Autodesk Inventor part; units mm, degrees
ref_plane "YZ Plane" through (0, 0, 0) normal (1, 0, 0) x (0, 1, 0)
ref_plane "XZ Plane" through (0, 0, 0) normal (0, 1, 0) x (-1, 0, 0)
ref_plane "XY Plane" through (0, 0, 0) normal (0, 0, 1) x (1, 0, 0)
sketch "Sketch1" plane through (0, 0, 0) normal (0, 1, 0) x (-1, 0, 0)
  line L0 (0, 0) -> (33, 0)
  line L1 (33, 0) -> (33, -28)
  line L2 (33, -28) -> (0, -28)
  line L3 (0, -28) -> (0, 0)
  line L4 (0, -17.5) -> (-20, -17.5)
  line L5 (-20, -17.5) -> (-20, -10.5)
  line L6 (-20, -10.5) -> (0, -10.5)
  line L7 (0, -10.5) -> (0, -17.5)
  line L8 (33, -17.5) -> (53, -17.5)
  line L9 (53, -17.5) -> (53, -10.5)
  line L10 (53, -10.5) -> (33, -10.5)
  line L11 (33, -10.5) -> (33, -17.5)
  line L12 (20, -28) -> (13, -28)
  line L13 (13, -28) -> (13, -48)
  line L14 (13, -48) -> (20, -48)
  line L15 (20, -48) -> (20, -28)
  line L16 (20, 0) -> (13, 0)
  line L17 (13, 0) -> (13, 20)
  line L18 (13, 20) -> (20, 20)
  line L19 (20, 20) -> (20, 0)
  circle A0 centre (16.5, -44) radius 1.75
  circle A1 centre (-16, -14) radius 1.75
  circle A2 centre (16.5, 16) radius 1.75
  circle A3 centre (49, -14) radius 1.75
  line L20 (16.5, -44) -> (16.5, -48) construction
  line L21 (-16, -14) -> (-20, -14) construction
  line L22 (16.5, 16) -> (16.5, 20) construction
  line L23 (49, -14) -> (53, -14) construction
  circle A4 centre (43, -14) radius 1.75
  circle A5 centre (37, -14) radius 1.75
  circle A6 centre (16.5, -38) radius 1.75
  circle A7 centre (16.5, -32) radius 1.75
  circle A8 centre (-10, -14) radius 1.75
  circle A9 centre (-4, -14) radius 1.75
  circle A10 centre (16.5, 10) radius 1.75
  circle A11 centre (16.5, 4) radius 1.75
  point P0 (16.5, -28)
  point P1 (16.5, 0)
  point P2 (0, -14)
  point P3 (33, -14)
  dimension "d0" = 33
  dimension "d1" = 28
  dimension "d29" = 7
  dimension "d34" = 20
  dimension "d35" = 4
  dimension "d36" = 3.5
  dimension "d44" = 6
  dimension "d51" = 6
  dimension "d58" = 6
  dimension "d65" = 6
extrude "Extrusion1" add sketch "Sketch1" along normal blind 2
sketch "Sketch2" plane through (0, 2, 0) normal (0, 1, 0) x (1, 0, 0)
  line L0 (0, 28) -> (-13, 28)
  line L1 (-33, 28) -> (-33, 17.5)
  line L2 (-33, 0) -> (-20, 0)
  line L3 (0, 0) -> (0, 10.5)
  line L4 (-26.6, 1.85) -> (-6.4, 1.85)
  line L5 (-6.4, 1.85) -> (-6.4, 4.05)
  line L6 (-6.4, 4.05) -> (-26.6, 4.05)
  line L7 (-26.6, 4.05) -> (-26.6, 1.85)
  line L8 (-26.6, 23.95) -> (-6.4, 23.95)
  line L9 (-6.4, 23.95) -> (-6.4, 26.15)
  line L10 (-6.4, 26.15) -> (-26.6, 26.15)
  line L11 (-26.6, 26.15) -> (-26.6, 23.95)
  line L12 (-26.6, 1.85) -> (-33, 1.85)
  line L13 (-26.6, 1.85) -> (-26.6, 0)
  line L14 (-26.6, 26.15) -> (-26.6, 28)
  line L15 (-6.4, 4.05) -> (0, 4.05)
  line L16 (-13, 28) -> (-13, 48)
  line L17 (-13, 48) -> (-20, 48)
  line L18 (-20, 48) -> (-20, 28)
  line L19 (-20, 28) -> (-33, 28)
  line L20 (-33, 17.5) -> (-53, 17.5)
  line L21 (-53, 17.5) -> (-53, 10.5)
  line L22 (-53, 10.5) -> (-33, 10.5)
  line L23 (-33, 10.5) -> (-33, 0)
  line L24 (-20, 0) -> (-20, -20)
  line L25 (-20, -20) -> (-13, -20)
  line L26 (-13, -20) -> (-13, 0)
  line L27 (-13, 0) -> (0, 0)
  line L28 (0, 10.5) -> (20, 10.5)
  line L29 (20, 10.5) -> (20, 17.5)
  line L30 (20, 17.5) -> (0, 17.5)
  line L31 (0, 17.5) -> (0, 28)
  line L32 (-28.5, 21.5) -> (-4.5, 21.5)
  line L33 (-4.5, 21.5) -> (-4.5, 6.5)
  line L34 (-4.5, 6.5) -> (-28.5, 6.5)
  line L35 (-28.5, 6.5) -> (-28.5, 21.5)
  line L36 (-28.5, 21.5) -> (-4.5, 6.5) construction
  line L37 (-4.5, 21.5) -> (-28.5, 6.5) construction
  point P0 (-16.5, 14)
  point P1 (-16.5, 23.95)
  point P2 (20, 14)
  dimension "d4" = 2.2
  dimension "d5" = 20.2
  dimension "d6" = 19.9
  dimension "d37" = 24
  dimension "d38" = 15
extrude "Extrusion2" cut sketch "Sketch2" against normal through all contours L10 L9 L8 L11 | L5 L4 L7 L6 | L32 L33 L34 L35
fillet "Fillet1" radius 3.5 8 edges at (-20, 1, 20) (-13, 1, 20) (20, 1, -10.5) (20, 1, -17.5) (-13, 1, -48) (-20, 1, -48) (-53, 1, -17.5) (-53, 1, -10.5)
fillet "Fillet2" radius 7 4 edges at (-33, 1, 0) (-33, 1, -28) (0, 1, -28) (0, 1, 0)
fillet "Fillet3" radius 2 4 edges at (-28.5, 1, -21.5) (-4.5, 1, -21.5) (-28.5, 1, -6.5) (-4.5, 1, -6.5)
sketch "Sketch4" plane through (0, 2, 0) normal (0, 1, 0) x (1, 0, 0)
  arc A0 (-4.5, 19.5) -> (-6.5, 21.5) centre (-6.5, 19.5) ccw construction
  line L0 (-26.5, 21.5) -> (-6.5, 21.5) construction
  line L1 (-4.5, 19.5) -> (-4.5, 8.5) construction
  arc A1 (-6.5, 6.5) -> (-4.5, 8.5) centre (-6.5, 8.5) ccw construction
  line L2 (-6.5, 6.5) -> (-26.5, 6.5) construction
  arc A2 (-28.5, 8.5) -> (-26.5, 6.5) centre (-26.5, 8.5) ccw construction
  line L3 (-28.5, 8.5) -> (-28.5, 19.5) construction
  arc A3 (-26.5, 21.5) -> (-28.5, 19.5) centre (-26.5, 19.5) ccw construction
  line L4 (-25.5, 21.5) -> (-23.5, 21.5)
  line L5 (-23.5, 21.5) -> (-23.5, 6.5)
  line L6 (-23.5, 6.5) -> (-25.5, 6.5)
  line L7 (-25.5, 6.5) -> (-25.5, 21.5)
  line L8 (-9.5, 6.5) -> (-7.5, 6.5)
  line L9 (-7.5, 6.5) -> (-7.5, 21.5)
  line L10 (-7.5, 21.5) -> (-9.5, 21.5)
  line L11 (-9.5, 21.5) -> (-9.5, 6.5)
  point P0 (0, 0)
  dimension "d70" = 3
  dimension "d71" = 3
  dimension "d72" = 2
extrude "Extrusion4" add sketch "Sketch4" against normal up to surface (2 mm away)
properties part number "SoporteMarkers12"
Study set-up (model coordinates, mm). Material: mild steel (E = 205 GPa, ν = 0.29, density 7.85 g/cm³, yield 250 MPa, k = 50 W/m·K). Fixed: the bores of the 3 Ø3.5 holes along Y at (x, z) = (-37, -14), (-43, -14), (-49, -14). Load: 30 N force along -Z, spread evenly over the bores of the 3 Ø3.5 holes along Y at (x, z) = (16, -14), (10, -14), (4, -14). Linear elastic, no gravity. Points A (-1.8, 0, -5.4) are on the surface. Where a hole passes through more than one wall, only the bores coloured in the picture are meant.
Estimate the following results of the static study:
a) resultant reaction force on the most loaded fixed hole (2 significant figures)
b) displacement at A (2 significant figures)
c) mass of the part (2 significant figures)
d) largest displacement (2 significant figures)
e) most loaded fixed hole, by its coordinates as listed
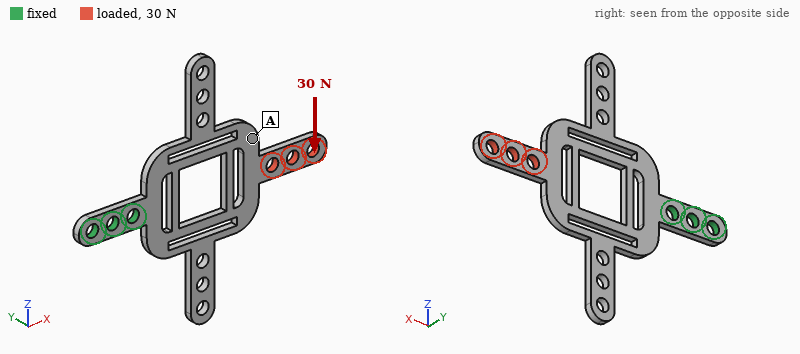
72 N
57 µm
14 g
87 µm
(-37, -14)
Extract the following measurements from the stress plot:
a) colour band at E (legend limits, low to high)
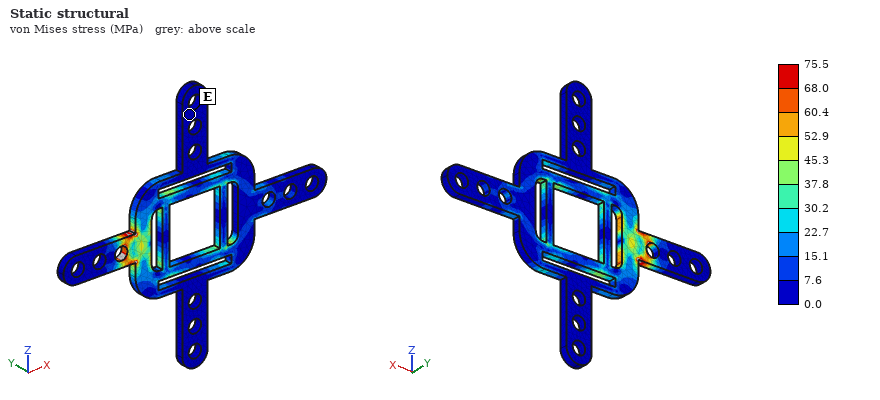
0.0 to 7.6 MPa
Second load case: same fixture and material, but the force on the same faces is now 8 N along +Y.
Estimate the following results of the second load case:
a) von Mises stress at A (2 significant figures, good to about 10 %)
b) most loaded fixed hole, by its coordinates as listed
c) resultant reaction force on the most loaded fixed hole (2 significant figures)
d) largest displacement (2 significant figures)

12 MPa
(-37, -14)
9.6 N
0.34 mm
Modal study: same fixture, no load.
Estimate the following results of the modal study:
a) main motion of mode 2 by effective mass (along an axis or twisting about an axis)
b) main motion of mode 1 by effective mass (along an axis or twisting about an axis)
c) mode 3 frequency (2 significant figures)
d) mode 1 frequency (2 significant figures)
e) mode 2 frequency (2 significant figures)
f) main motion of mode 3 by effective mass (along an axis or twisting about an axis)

twisting about X
along Y
1400 Hz
510 Hz
890 Hz
along Z
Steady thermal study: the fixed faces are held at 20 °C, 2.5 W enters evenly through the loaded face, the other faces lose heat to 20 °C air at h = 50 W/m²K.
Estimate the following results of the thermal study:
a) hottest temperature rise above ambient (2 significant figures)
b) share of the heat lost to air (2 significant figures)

70 K
87 %
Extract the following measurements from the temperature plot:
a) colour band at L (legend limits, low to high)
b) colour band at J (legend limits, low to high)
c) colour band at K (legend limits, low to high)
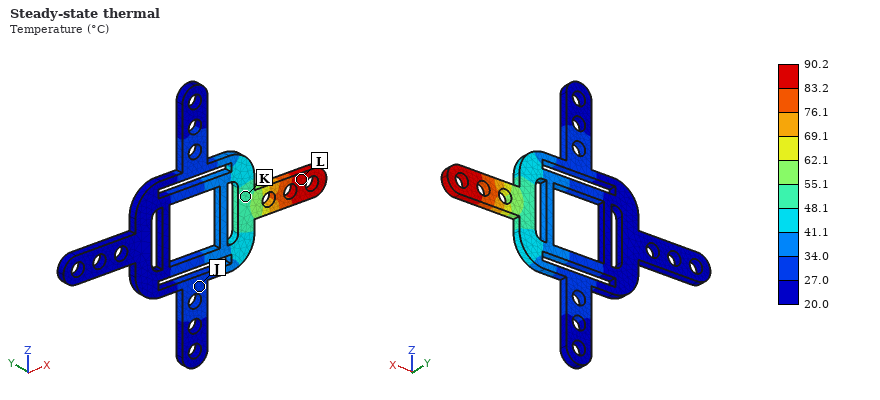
83.2 to 90.2 °C
27.0 to 34.0 °C
48.1 to 55.1 °C
